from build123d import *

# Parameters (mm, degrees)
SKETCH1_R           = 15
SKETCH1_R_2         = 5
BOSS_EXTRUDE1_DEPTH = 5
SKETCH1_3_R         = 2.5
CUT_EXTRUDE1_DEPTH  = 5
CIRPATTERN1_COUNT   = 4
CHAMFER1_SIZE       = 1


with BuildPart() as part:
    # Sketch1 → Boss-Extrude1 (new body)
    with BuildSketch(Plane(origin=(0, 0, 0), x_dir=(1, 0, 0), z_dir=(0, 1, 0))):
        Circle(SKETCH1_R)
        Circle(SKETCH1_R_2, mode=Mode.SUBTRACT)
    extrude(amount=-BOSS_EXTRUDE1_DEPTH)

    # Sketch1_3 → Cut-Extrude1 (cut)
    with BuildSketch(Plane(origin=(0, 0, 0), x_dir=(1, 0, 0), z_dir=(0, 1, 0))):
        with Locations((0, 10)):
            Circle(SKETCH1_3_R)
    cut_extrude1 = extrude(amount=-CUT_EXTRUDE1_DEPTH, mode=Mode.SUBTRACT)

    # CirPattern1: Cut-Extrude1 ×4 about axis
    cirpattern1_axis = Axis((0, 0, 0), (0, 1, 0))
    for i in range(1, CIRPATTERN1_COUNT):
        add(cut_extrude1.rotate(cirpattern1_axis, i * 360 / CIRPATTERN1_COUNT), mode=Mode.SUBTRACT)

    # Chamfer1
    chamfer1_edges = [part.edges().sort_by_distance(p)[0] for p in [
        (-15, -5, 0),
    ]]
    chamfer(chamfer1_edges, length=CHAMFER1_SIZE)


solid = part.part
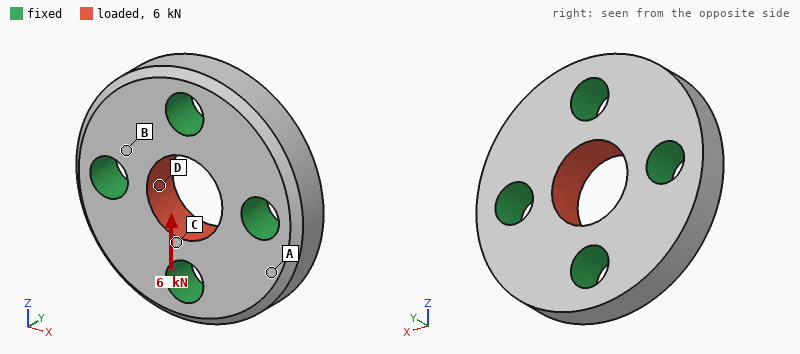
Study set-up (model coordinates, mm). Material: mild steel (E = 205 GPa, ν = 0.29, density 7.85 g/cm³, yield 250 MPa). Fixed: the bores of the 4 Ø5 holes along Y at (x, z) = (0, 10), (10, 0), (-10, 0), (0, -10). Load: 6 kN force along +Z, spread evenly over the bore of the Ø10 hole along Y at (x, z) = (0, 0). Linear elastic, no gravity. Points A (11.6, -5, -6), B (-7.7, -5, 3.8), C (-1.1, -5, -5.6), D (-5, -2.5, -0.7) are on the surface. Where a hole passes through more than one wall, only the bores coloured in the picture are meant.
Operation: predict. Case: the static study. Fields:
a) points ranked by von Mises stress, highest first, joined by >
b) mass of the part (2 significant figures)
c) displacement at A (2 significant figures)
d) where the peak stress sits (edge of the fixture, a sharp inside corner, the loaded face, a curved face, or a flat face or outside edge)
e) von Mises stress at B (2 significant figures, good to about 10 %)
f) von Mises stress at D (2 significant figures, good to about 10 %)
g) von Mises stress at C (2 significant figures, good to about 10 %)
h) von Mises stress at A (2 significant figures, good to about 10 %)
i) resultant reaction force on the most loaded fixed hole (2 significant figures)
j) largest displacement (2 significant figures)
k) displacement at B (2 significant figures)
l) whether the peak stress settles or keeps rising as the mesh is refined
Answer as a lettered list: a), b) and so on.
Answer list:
a) D > C > B > A
b) 21 g
c) 0.23 µm
d) edge of the fixture
e) 20 MPa
f) 66 MPa
g) 46 MPa
h) 7.8 MPa
i) 1.8 kN
j) 1.2 µm
k) 0.40 µm
l) keeps rising
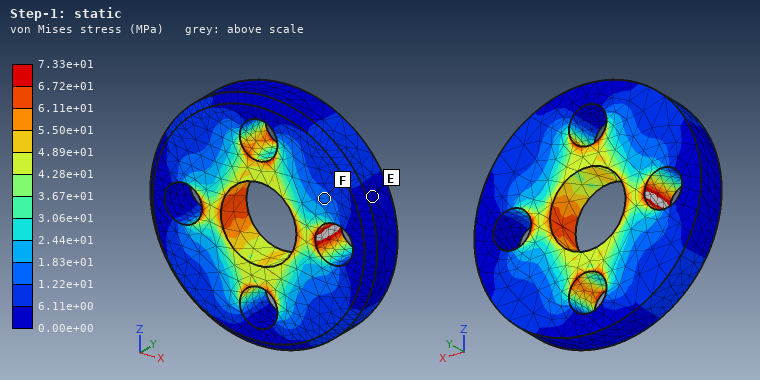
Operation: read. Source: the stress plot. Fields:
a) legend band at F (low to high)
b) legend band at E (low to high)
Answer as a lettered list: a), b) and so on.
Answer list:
a) 1.22e+01 to 1.83e+01 MPa
b) 0.00e+00 to 6.11e+00 MPa
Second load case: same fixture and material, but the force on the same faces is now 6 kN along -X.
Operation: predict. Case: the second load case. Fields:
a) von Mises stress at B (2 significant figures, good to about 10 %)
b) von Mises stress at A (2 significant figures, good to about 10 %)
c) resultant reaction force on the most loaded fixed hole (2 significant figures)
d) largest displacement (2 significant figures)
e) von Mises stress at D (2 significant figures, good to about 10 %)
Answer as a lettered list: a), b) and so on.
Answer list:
a) 24 MPa
b) 8.7 MPa
c) 1.8 kN
d) 1.2 µm
e) 51 MPa
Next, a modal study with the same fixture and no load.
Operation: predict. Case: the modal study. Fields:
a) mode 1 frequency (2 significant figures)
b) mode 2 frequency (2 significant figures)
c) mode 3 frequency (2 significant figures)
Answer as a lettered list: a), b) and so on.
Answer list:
a) 72 kHz
b) 73 kHz
c) 73 kHz
